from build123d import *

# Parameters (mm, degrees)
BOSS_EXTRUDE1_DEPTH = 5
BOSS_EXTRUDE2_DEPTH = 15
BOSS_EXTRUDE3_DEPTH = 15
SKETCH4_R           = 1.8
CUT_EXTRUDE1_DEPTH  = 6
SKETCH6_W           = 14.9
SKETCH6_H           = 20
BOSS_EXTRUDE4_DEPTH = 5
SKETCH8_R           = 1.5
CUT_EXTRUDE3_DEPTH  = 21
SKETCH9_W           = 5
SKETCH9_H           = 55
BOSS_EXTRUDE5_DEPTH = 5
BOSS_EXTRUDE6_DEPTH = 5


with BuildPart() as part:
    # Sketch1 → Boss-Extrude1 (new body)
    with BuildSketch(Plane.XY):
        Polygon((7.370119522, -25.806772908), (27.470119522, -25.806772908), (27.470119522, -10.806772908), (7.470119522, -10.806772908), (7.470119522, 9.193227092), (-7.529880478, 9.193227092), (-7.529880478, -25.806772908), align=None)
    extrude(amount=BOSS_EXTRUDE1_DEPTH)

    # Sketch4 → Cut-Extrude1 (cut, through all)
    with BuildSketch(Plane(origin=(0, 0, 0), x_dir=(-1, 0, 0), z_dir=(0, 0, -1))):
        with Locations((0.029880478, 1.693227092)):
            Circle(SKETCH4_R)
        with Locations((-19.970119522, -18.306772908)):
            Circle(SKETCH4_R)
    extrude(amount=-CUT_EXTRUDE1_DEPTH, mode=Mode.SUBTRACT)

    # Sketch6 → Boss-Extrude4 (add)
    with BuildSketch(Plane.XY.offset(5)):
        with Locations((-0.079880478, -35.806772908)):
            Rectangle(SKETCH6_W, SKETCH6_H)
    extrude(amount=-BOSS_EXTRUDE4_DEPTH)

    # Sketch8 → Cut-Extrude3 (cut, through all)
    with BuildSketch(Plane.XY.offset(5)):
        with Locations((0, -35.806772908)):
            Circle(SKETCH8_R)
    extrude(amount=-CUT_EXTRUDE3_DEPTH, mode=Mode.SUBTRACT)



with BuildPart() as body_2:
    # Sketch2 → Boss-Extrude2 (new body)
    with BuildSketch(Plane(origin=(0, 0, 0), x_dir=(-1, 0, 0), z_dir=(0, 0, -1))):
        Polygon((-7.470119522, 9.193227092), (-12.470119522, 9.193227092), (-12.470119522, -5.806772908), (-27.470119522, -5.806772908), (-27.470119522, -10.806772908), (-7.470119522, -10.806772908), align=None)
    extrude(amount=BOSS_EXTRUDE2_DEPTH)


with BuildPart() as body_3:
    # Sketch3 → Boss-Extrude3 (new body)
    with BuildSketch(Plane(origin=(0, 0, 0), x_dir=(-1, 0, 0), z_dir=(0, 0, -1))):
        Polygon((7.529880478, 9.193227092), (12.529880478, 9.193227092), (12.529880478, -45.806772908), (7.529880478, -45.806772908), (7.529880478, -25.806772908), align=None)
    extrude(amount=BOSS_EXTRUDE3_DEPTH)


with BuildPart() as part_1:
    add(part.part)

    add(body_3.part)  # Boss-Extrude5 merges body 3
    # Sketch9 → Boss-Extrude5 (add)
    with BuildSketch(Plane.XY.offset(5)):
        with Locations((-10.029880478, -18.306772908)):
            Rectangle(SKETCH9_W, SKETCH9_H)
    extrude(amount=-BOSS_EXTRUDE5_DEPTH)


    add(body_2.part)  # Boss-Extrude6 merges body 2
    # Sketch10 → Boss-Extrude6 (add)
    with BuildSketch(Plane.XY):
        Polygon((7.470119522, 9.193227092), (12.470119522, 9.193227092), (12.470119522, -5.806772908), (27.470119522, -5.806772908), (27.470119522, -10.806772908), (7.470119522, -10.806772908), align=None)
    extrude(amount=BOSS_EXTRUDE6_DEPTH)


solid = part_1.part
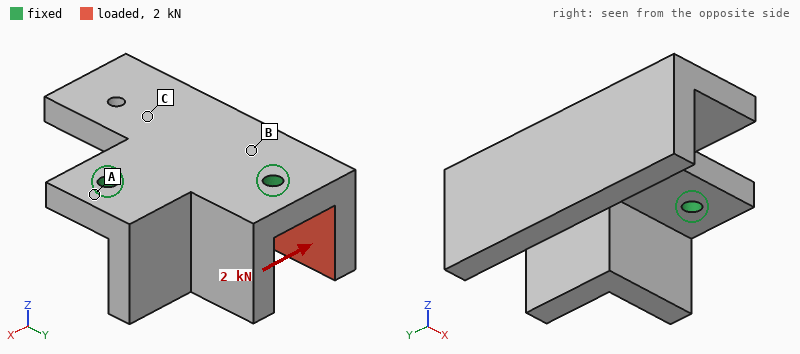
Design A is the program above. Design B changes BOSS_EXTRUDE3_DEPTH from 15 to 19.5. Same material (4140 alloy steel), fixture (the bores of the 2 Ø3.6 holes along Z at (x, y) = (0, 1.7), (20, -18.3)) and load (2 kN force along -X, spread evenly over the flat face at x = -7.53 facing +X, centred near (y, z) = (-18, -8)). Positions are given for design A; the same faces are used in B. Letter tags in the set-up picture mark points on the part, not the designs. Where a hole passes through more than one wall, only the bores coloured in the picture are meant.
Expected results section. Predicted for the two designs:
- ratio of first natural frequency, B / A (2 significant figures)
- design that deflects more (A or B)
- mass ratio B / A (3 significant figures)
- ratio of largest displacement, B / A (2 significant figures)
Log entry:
0.89
B
1.09
1.4
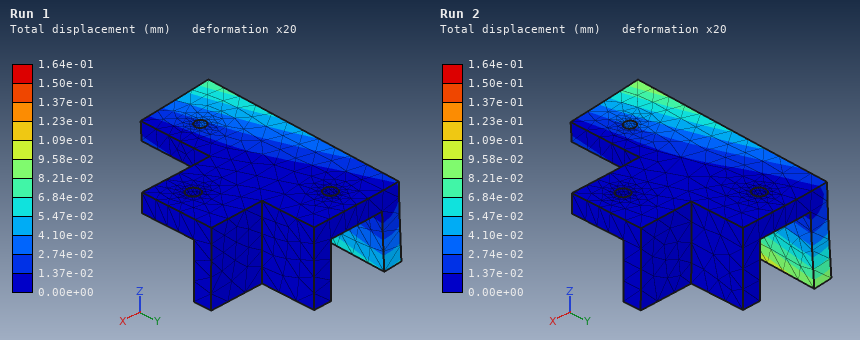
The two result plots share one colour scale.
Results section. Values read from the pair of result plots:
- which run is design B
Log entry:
Run 2
